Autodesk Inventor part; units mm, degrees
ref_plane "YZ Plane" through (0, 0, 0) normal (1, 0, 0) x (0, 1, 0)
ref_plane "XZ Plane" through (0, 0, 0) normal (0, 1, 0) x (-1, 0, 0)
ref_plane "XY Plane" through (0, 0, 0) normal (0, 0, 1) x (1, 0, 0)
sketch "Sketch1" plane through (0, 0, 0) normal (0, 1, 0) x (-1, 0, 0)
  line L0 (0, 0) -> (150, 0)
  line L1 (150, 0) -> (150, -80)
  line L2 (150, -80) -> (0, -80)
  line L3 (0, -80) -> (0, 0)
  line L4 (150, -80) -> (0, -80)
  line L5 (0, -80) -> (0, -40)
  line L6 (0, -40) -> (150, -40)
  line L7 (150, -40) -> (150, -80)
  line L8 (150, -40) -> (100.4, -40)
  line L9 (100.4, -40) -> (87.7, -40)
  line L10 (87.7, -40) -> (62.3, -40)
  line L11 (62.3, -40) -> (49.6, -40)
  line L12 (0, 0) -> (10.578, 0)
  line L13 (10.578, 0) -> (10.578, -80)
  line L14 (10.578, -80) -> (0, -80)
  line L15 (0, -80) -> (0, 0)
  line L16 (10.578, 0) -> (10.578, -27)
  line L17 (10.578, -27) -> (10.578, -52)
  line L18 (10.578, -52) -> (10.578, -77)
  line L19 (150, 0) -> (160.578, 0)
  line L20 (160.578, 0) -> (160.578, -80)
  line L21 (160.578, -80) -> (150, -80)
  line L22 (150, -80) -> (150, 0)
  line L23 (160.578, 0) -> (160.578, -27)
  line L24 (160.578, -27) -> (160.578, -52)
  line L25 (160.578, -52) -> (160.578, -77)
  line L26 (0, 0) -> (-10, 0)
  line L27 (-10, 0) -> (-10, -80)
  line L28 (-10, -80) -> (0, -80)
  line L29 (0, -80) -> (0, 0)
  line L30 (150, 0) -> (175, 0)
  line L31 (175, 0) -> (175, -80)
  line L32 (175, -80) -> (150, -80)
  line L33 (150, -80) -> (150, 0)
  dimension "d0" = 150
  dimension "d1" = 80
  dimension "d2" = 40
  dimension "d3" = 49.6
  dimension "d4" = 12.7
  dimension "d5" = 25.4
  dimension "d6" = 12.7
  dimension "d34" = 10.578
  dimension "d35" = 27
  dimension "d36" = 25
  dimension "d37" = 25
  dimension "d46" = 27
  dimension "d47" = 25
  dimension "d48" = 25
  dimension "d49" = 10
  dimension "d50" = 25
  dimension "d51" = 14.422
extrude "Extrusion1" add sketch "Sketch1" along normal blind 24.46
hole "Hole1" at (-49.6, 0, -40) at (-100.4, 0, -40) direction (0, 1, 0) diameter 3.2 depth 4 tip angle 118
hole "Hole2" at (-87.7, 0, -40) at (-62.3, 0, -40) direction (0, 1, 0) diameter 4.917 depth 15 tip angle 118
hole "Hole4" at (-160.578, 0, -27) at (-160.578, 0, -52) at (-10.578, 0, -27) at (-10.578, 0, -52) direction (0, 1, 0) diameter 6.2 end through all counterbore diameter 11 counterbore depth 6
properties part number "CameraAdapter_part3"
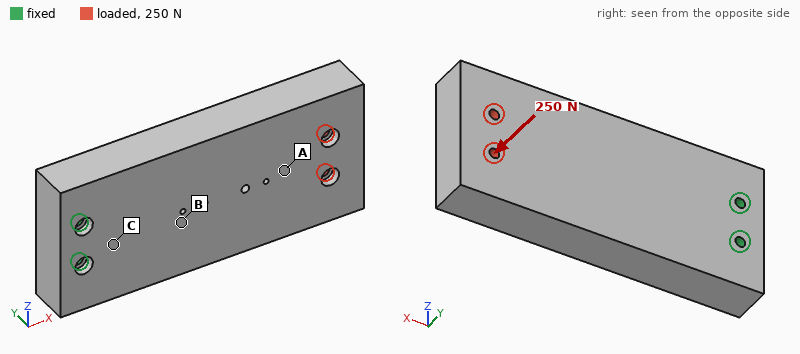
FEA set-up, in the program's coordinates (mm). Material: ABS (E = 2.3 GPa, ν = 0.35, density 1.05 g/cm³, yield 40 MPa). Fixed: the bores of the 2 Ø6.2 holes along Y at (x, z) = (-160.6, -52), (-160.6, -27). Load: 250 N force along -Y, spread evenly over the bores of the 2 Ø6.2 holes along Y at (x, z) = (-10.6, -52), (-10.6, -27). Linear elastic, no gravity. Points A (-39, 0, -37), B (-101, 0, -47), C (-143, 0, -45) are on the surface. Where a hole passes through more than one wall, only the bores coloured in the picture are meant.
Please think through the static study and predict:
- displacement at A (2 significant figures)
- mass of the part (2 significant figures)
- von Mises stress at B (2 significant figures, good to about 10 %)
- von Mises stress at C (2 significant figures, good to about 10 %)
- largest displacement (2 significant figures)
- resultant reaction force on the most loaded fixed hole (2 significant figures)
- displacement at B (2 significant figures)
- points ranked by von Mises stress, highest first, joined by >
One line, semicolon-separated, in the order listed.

1.3 mm; 370 g; 2.7 MPa; 4.1 MPa; 2.1 mm; 140 N; 0.48 mm; C > B > A
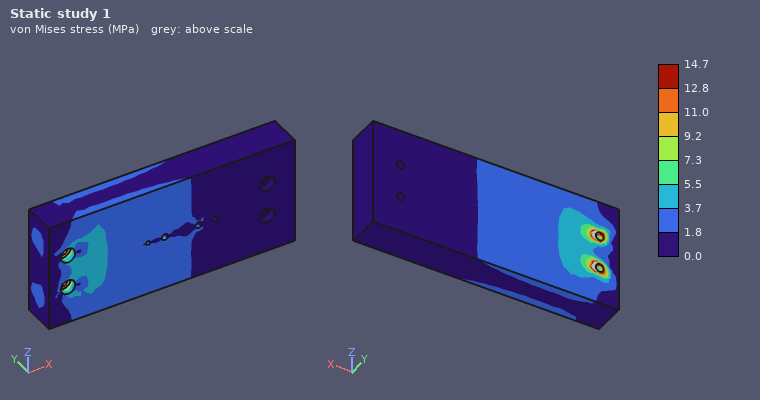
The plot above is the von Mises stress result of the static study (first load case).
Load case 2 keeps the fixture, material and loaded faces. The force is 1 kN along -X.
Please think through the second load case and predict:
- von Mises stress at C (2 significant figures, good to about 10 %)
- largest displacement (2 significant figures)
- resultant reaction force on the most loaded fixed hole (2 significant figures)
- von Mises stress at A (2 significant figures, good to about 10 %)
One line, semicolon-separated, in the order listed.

0.30 MPa; 0.19 mm; 500 N; 0.31 MPa
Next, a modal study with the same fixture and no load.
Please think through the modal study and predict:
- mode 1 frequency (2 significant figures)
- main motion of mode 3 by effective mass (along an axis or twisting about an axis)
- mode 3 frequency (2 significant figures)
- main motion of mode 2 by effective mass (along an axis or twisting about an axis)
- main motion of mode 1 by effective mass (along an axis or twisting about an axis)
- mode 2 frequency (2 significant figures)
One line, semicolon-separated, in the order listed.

170 Hz; twisting about X; 680 Hz; along Z; along Y; 350 Hz
